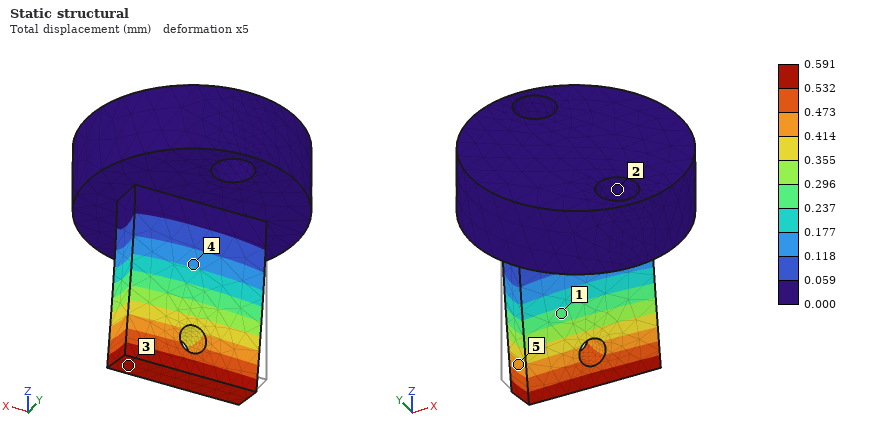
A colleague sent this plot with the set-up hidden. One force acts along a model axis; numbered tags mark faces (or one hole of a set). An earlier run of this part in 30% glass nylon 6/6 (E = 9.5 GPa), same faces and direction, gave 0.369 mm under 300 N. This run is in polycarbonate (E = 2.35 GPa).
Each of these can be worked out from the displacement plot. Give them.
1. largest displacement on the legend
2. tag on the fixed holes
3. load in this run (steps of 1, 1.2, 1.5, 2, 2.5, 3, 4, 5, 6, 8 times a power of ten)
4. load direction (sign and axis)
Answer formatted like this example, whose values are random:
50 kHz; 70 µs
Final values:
0.591 mm; 2; 120 N; -Y
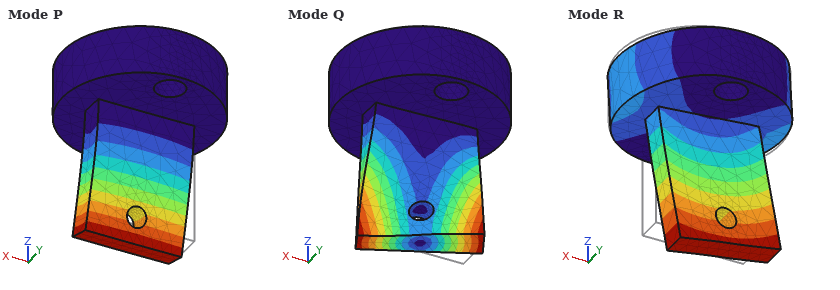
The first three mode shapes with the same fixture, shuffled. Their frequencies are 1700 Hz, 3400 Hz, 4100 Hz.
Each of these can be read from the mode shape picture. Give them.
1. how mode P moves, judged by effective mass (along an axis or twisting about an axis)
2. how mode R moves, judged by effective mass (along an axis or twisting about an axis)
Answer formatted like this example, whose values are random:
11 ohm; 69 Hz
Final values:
along Y; along X
